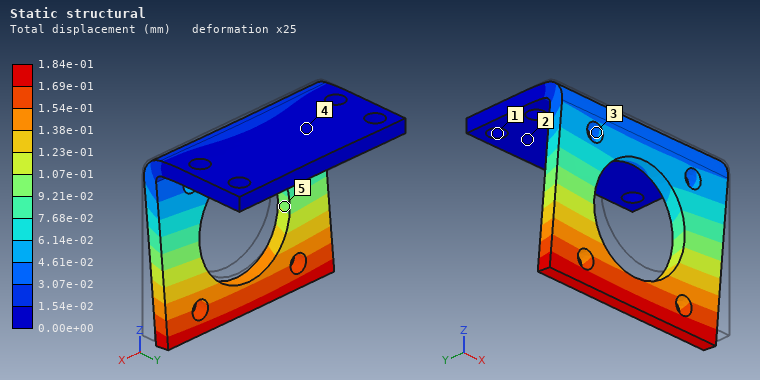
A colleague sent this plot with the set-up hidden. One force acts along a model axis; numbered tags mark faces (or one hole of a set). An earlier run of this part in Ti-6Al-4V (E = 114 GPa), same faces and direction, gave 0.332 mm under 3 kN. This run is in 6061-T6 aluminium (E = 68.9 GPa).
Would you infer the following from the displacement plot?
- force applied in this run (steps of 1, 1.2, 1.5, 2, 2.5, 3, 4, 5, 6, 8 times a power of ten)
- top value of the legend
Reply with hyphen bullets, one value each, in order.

- 1 kN
- 1.84e-01 mm
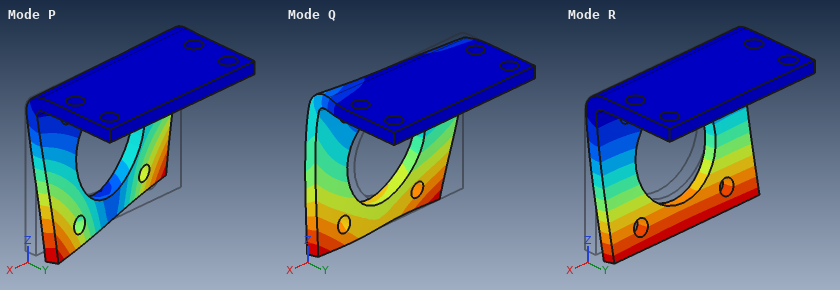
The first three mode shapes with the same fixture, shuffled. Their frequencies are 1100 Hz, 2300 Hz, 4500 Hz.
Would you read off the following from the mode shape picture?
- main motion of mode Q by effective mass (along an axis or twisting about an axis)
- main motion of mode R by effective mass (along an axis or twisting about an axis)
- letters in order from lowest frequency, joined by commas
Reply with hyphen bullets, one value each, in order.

- along X
- along Y
- R, P, Q
